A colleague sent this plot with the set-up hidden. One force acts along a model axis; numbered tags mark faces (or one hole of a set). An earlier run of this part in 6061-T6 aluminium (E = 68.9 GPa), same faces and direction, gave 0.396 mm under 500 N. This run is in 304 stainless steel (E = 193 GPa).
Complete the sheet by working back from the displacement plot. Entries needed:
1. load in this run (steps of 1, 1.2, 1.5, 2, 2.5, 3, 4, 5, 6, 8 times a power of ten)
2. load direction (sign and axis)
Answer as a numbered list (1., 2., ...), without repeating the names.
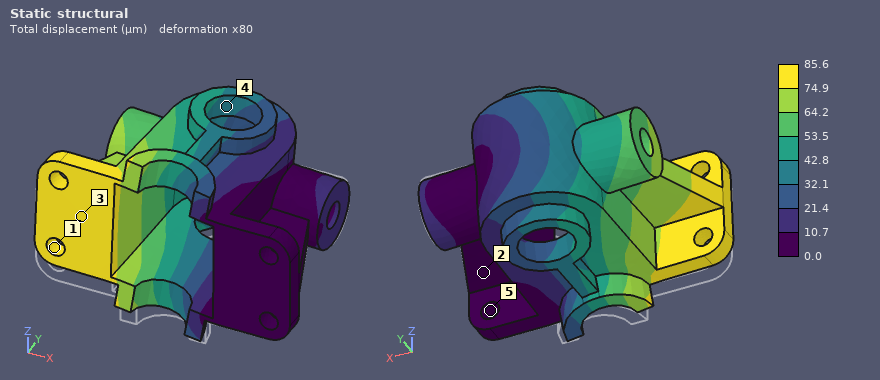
1. 300 N
2. +Z
